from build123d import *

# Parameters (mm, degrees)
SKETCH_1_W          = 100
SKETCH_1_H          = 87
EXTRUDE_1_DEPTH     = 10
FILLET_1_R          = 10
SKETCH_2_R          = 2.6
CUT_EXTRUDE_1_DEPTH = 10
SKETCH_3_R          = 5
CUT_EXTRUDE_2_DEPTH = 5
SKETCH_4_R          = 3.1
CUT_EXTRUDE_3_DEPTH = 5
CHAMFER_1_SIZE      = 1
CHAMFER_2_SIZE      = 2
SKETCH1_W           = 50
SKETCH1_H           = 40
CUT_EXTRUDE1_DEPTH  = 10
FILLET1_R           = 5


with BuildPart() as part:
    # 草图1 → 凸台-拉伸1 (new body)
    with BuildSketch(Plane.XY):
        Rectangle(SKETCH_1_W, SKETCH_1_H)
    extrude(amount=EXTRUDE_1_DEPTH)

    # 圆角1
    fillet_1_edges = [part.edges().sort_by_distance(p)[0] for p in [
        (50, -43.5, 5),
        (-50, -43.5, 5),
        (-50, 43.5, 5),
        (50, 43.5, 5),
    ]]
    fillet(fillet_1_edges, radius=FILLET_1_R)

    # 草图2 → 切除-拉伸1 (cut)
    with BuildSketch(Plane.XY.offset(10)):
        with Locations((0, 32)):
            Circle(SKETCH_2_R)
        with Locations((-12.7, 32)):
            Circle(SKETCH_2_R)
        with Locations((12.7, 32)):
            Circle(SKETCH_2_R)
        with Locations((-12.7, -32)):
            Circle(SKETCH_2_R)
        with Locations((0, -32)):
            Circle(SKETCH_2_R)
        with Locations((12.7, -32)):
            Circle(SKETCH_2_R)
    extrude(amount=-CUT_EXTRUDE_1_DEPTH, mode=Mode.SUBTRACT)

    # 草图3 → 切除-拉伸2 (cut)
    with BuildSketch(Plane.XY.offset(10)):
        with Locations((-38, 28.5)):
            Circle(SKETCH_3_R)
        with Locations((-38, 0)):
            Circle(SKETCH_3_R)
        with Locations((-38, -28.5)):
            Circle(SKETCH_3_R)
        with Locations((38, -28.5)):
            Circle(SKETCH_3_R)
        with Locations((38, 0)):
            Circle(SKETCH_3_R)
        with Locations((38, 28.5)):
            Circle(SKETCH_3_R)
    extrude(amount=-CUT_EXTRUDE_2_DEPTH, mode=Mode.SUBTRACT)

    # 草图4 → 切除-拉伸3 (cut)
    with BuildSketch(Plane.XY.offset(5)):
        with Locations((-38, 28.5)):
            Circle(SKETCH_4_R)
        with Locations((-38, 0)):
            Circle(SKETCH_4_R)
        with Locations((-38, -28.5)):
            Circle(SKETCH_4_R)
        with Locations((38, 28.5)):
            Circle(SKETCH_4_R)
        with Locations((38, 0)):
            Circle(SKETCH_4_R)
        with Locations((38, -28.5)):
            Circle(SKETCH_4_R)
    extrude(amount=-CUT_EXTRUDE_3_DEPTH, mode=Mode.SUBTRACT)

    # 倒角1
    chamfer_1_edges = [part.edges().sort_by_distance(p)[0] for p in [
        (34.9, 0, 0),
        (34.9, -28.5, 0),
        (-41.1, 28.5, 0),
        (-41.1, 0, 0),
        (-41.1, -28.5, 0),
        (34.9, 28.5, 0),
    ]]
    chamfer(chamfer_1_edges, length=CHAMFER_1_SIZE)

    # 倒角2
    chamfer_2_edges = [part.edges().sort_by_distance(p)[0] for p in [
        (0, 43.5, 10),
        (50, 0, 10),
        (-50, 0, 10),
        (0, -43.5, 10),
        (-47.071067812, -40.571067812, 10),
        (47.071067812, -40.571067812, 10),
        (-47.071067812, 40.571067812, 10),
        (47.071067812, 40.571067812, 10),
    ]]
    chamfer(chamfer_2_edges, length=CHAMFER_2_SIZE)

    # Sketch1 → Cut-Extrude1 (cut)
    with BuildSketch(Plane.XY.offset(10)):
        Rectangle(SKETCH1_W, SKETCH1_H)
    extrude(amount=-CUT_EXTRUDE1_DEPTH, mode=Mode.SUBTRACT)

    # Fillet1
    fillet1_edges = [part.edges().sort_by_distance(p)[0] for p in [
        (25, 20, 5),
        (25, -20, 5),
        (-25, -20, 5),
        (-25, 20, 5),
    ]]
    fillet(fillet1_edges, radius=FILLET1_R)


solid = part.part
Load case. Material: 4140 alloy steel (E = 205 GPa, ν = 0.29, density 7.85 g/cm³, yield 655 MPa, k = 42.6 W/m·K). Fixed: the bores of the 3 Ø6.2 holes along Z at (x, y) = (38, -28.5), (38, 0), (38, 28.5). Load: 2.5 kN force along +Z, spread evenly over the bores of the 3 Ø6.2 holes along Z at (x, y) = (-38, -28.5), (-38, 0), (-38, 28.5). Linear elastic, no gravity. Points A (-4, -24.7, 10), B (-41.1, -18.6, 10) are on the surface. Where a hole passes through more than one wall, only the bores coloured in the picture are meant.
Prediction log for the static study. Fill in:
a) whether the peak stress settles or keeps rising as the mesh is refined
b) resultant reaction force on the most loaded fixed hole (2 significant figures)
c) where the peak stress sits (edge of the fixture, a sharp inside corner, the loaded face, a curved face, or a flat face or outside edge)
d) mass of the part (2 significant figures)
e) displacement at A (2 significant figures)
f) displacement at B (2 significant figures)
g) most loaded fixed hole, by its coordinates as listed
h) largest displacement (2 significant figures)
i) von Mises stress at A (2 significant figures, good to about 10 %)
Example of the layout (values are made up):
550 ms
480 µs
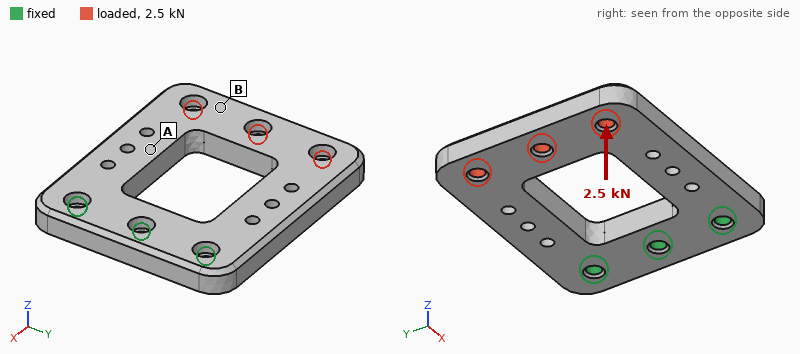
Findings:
keeps rising
1.5 kN
edge of the fixture
480 g
0.28 mm
0.70 mm
(38, 0)
0.81 mm
140 MPa
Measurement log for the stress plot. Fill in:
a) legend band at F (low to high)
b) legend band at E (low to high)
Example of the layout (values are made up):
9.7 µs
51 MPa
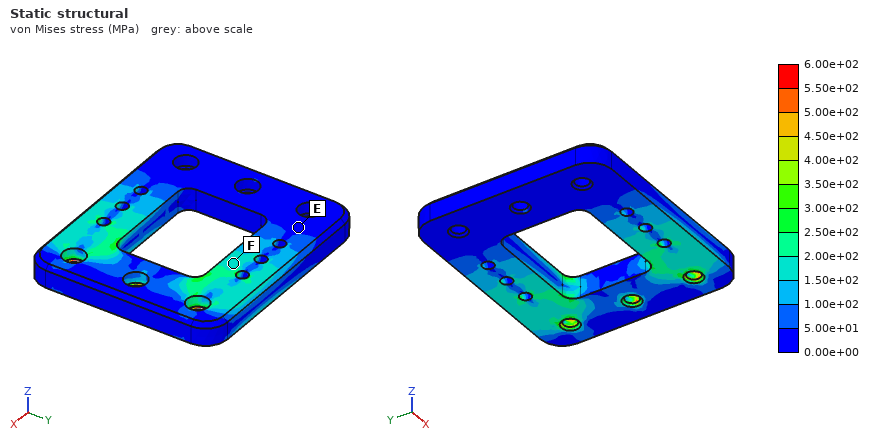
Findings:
1.50e+02 to 2.00e+02 MPa
0.00e+00 to 5.00e+01 MPa
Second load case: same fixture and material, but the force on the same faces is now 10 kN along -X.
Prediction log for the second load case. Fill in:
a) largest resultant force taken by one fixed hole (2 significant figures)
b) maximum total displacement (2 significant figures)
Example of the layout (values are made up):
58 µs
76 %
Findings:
5.0 kN
92 µm
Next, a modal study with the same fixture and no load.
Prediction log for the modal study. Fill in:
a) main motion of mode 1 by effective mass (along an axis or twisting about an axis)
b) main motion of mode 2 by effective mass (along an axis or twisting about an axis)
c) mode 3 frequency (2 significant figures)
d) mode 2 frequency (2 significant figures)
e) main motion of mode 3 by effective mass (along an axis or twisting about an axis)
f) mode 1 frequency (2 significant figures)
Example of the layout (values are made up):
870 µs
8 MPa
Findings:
along Z
twisting about X
2900 Hz
1800 Hz
along Y
720 Hz
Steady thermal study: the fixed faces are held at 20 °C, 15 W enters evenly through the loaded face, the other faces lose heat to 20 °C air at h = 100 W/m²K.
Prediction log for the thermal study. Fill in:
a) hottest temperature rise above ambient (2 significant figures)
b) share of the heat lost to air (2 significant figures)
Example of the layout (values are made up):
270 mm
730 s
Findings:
20 K
88 %
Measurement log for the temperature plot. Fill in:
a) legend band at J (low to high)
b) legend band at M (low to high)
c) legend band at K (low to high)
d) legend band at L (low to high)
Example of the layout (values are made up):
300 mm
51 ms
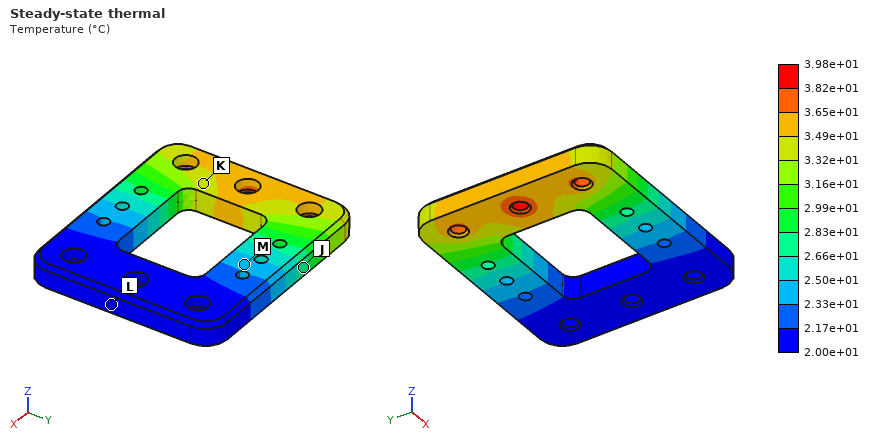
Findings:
2.66e+01 to 2.83e+01 °C
2.33e+01 to 2.50e+01 °C
3.32e+01 to 3.49e+01 °C
2.00e+01 to 2.17e+01 °C
